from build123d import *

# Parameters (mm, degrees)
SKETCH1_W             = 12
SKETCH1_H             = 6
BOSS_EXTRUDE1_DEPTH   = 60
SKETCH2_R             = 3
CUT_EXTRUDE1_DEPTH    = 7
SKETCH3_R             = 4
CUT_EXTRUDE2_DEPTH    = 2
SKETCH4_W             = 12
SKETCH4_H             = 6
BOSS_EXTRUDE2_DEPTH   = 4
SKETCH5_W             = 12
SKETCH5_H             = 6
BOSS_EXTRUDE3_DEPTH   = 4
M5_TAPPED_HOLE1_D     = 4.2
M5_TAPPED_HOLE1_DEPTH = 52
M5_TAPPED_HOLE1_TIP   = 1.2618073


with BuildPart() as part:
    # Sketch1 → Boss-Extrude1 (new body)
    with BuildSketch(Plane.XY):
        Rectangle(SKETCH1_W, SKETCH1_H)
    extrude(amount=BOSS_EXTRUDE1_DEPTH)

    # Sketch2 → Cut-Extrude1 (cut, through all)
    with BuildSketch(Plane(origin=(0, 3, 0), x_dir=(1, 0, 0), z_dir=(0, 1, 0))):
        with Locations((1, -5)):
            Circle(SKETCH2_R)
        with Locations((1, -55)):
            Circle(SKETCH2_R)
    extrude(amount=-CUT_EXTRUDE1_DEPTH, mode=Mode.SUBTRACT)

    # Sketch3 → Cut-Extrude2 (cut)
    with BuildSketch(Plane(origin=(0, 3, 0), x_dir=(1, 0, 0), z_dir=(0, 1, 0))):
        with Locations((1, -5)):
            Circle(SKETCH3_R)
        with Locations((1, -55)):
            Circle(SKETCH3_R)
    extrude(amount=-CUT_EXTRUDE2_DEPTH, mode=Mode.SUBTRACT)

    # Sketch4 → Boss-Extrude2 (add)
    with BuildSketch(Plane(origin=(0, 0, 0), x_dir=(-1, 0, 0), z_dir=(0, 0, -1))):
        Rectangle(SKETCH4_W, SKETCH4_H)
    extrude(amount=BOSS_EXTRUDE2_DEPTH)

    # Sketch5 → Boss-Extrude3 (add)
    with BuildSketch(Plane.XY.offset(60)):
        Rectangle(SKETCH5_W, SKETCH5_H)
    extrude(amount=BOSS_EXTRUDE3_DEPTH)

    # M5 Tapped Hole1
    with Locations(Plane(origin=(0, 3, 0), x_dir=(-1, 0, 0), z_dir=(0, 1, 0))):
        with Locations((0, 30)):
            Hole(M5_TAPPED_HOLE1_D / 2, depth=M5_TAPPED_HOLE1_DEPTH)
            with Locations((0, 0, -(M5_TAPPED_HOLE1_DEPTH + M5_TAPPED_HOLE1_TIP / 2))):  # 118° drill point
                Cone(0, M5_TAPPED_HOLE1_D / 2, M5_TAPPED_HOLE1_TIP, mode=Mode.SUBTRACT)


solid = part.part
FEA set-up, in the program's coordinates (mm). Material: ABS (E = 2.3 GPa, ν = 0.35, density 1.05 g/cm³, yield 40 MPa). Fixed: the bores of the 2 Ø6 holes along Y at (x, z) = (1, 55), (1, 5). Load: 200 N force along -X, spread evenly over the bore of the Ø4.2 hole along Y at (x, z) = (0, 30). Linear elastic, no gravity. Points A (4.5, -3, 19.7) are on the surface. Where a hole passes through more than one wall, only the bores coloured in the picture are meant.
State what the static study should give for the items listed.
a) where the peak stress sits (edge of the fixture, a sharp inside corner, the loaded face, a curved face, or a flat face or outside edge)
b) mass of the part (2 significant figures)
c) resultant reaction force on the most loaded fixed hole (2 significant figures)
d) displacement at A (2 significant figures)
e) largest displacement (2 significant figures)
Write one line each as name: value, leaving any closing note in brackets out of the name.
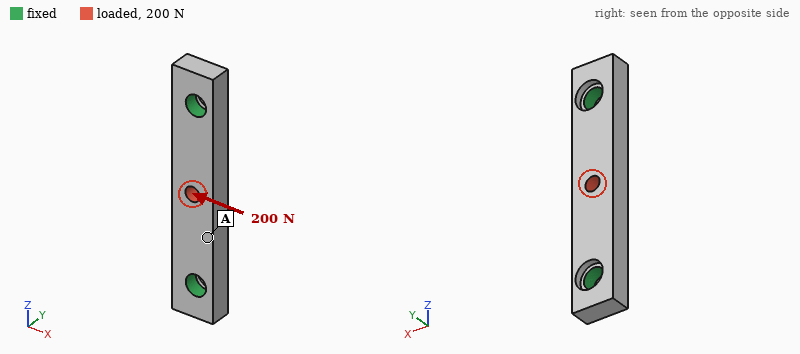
where the peak stress sits: edge of the fixture
mass of the part: 4.6 g
resultant reaction force on the most loaded fixed hole: 100 N
displacement at A: 0.079 mm
largest displacement: 0.13 mm
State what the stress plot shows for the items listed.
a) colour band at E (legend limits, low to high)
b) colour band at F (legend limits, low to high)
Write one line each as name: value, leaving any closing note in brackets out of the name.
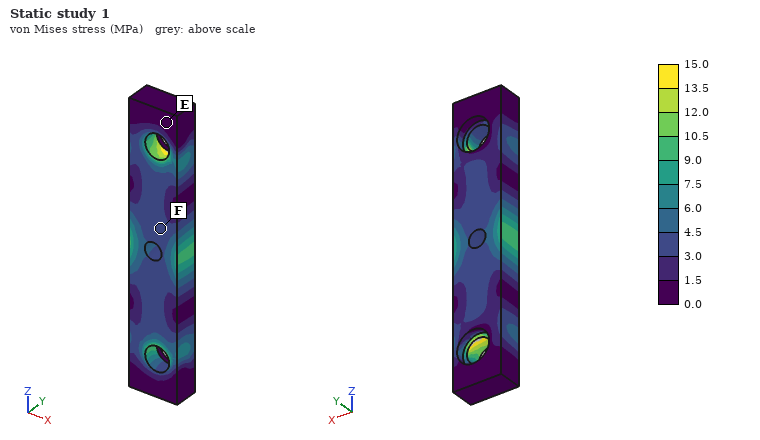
colour band at E: 0.0 to 1.5 MPa
colour band at F: 3.0 to 4.5 MPa
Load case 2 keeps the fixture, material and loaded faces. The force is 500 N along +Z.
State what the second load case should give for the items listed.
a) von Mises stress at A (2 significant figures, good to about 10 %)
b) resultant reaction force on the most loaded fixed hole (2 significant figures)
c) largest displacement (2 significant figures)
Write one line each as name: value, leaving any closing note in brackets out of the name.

von Mises stress at A: 4.3 MPa
resultant reaction force on the most loaded fixed hole: 250 N
largest displacement: 45 µm
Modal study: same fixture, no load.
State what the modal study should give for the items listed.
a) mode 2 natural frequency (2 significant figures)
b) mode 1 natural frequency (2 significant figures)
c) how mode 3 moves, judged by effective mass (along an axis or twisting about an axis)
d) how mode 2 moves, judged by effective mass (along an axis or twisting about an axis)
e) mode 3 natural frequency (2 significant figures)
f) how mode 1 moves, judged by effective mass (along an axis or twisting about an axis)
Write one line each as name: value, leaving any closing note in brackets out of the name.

mode 2 natural frequency: 5300 Hz
mode 1 natural frequency: 3300 Hz
how mode 3 moves, judged by effective mass: twisting about Z
how mode 2 moves, judged by effective mass: along X
mode 3 natural frequency: 6700 Hz
how mode 1 moves, judged by effective mass: along Y
